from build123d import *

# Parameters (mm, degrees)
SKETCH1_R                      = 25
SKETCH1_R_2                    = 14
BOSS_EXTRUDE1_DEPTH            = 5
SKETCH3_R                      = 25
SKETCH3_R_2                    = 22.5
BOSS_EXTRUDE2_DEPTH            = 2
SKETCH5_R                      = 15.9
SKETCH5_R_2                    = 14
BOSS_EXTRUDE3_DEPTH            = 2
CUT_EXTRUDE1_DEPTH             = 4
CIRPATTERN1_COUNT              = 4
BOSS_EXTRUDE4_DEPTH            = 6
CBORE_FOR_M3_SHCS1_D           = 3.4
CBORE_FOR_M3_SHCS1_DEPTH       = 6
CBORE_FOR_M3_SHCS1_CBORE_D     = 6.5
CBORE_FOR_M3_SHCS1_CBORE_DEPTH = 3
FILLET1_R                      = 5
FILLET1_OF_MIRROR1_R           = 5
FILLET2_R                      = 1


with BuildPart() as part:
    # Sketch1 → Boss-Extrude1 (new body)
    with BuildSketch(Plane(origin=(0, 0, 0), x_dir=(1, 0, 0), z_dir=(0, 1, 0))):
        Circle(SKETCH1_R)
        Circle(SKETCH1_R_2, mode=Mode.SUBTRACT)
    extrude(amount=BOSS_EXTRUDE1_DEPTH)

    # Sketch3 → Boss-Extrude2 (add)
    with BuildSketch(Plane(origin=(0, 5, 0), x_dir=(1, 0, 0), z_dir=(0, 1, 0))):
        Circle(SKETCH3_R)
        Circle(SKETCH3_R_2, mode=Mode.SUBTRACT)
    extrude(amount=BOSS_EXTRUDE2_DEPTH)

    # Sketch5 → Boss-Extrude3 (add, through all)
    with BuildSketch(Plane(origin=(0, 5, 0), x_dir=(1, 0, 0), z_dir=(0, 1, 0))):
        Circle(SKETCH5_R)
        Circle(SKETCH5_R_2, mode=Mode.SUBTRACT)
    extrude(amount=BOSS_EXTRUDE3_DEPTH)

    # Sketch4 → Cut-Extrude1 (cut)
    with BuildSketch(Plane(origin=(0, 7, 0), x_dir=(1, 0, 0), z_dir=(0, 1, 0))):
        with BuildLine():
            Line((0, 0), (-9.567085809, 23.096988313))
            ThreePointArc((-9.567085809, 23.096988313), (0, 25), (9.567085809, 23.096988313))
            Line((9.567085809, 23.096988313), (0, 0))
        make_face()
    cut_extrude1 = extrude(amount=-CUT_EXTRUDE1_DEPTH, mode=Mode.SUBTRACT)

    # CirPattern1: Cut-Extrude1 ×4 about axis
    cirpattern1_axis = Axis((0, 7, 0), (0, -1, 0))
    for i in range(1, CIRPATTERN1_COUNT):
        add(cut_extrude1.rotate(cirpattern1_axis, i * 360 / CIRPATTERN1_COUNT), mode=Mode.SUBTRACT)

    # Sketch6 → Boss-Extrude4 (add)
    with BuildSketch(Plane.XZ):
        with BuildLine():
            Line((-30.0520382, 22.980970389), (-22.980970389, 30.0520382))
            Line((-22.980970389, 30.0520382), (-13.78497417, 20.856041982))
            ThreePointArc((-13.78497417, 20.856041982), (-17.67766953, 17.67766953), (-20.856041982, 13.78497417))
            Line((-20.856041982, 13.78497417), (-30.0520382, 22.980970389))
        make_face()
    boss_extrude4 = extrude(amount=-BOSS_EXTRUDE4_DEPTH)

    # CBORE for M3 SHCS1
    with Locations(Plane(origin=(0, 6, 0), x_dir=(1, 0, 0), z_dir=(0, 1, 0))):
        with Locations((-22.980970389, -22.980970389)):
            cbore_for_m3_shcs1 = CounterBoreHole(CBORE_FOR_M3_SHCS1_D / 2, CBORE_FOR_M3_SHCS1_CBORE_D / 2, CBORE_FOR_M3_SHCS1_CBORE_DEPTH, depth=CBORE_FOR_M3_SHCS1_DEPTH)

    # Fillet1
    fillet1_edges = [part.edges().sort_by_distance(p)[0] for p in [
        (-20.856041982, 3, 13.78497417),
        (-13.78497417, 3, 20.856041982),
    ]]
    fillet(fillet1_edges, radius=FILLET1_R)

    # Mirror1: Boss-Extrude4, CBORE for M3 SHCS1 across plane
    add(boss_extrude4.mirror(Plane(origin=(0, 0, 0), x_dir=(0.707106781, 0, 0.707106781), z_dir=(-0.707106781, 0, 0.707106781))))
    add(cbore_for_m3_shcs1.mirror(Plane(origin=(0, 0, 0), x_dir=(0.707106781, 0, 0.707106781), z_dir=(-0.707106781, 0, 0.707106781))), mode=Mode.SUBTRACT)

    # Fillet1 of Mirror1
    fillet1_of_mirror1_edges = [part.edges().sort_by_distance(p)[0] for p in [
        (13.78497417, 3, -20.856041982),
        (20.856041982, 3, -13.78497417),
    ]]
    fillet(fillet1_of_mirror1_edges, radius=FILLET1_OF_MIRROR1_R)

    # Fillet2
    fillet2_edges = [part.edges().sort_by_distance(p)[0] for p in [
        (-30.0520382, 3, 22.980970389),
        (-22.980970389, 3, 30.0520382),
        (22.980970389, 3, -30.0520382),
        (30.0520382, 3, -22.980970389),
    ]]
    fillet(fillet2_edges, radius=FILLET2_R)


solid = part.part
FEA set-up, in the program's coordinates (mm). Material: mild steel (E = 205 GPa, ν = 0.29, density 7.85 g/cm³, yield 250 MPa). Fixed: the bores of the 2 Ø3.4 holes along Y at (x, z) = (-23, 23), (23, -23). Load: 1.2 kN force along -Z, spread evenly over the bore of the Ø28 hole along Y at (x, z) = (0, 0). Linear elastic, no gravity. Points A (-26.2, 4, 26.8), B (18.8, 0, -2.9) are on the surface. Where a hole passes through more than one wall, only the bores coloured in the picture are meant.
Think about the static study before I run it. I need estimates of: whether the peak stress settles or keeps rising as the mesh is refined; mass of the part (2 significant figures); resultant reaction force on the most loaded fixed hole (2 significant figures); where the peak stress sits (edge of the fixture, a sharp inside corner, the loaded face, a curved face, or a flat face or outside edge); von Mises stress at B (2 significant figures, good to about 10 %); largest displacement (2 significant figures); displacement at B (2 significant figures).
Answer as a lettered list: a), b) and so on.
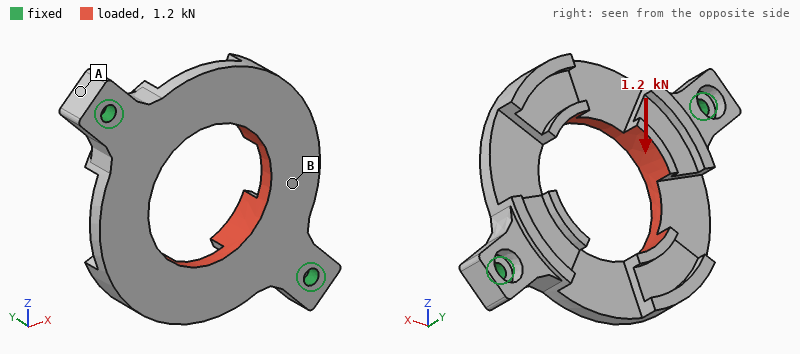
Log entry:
a) keeps rising
b) 57 g
c) 600 N
d) edge of the fixture
e) 18 MPa
f) 11 µm
g) 2.8 µm
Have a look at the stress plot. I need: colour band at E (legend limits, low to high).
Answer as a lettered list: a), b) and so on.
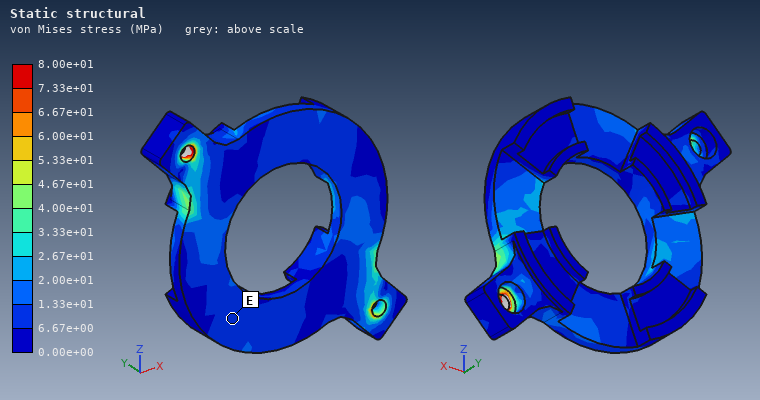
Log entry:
a) 6.67e+00 to 1.33e+01 MPa
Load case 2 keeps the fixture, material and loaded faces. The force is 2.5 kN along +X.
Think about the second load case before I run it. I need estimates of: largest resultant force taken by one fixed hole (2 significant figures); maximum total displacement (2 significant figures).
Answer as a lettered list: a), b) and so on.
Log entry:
a) 1.3 kN
b) 22 µm
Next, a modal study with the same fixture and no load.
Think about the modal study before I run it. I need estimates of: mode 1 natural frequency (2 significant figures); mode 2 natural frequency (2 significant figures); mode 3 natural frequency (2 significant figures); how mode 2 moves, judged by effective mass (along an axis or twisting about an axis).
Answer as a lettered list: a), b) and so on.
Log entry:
a) 2700 Hz
b) 3000 Hz
c) 7400 Hz
d) along Y
